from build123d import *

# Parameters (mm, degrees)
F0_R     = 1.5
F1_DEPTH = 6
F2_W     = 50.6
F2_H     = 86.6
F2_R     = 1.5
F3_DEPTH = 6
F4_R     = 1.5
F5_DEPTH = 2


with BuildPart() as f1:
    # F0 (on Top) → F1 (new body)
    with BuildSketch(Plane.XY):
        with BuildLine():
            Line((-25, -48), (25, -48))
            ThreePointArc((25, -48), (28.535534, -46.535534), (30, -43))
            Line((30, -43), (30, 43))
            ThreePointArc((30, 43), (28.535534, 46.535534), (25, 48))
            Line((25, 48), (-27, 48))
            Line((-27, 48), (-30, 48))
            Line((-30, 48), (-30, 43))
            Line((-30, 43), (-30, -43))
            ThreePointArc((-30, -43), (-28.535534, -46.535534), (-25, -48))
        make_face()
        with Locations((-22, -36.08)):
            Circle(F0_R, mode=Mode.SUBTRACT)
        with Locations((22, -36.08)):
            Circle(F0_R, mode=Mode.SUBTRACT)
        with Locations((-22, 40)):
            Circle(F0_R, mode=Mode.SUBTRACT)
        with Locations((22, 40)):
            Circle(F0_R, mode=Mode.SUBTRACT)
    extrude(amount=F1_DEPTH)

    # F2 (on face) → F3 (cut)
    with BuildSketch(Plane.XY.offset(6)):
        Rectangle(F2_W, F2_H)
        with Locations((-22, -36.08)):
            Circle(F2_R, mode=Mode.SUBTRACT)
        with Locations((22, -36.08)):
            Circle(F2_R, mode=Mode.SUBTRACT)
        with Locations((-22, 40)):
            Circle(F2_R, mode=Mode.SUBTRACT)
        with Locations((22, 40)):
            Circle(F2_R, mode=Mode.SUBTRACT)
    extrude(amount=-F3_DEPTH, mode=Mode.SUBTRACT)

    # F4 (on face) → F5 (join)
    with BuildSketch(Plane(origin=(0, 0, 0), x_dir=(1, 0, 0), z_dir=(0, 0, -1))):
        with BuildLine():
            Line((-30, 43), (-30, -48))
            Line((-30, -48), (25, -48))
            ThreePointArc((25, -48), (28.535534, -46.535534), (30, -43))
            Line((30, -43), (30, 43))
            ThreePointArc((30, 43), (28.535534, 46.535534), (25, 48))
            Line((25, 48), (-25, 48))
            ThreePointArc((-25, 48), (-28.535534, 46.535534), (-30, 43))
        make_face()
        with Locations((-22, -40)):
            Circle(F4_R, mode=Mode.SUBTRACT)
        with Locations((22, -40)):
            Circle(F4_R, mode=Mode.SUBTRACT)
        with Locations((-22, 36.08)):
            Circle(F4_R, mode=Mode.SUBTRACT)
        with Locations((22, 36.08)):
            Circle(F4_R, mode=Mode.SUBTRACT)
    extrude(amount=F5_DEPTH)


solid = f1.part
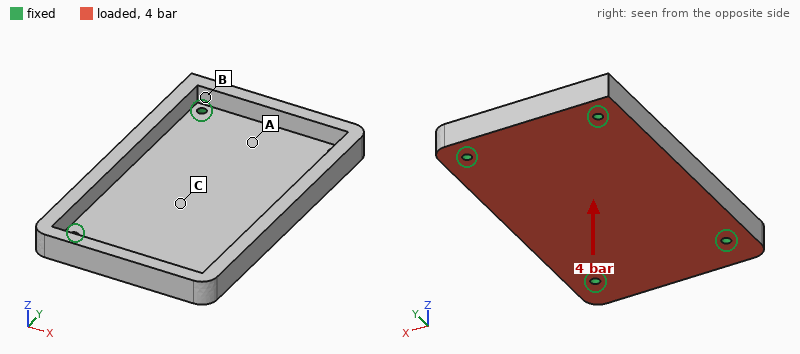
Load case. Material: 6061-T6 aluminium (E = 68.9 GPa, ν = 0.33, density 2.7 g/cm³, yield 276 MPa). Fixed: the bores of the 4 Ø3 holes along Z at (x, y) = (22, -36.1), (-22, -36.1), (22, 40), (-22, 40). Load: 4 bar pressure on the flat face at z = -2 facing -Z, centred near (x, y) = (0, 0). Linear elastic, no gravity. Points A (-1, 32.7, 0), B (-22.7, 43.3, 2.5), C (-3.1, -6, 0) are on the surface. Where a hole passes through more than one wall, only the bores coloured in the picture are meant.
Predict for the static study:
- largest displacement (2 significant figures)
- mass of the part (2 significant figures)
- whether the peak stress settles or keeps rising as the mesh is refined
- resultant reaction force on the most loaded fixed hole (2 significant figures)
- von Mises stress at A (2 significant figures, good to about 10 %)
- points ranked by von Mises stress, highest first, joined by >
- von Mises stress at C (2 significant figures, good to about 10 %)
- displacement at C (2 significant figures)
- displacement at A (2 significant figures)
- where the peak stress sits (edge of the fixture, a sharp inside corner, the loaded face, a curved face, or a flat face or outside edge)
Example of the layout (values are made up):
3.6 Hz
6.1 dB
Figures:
0.33 mm
53 g
keeps rising
750 N
34 MPa
C > A > B
66 MPa
0.31 mm
0.11 mm
edge of the fixture
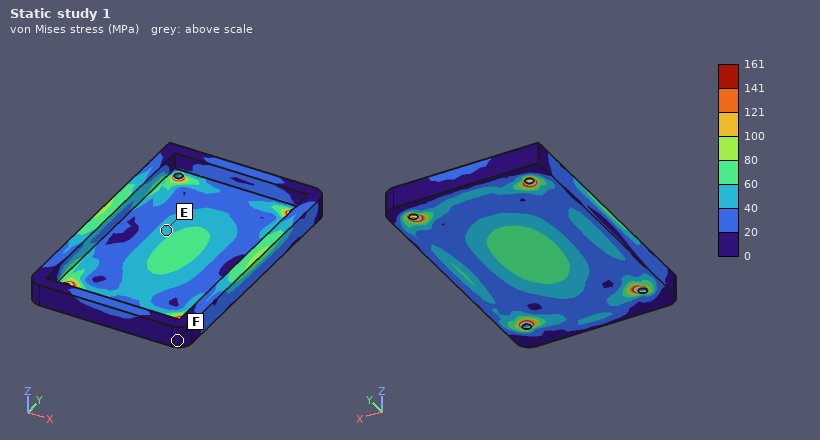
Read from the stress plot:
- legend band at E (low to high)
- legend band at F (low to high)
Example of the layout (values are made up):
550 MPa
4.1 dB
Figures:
40 to 60 MPa
0 to 20 MPa
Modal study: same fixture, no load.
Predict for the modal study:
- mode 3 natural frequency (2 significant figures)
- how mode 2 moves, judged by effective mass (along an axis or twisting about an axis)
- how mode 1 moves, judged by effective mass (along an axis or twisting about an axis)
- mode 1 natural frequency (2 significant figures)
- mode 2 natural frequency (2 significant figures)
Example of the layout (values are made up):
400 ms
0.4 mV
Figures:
4800 Hz
twisting about Y
along Z
2900 Hz
4300 Hz
